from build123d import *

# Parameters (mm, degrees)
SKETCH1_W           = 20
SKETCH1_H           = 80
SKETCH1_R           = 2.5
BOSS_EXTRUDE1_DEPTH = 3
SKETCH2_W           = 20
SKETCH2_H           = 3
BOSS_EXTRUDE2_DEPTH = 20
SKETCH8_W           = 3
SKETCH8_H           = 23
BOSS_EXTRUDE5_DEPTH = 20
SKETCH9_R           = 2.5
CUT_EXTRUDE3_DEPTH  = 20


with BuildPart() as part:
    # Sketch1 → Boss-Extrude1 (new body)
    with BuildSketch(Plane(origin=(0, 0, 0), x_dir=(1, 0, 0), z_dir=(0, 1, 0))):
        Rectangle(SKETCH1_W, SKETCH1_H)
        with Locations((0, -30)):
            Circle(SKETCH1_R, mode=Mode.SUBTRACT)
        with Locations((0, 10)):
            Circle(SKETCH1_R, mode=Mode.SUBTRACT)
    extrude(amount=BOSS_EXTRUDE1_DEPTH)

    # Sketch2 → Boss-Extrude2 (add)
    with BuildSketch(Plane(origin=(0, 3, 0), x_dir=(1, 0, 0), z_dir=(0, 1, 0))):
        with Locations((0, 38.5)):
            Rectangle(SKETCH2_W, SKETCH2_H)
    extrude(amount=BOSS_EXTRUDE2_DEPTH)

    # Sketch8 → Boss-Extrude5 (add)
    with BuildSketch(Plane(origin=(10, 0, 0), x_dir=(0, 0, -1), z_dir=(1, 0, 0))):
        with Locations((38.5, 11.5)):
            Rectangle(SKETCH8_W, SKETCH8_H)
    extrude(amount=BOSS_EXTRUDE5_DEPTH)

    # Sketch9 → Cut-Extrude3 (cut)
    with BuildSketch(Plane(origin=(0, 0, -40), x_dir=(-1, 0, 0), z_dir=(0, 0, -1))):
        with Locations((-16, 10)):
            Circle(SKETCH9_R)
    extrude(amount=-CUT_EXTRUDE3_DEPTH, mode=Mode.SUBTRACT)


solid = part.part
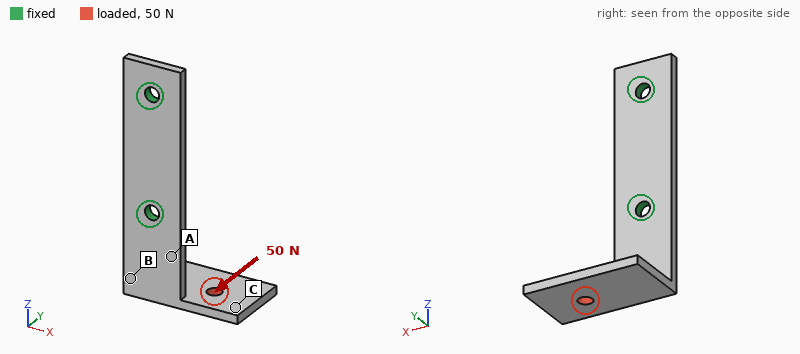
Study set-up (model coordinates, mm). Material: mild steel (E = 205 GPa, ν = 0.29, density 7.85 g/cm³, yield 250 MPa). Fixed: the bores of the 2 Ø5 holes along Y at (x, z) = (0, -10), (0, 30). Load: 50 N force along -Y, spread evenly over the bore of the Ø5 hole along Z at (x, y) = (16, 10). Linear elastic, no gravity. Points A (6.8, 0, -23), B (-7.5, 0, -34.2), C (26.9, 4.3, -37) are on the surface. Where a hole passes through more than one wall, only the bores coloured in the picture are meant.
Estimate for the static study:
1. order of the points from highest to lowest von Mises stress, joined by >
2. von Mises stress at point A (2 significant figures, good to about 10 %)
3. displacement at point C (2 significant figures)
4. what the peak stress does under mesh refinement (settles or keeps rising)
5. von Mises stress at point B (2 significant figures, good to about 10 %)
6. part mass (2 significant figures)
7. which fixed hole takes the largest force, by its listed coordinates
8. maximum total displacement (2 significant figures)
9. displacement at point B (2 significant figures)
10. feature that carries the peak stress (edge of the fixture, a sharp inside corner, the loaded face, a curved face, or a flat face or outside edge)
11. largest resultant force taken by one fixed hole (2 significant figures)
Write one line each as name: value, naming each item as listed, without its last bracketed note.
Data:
order of the points from highest to lowest von Mises stress, joined by >: A > B > C
von Mises stress at point A: 34 MPa
displacement at point C: 0.074 mm
what the peak stress does under mesh refinement: keeps rising
von Mises stress at point B: 20 MPa
part mass: 57 g
which fixed hole takes the largest force, by its listed coordinates: (0, -10)
maximum total displacement: 0.10 mm
displacement at point B: 0.019 mm
feature that carries the peak stress: edge of the fixture
largest resultant force taken by one fixed hole: 52 N
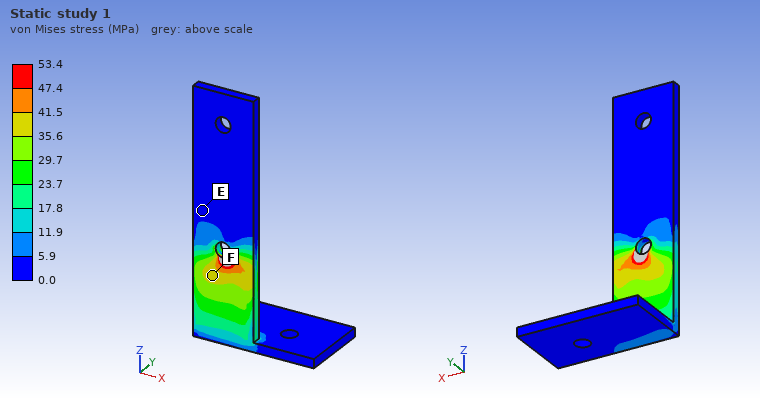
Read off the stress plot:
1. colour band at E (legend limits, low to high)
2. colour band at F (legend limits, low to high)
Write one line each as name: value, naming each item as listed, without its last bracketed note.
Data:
colour band at E: 0.0 to 5.9 MPa
colour band at F: 35.6 to 41.5 MPa
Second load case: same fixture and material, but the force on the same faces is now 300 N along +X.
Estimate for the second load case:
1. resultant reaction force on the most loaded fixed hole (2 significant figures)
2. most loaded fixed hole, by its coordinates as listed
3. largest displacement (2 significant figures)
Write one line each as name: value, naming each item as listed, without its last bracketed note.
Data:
resultant reaction force on the most loaded fixed hole: 430 N
most loaded fixed hole, by its coordinates as listed: (0, -10)
largest displacement: 0.18 mm
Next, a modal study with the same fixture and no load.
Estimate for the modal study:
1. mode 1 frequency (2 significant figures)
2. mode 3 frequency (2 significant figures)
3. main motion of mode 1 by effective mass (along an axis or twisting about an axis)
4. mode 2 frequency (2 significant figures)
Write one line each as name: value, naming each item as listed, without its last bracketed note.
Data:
mode 1 frequency: 920 Hz
mode 3 frequency: 2700 Hz
main motion of mode 1 by effective mass: along Y
mode 2 frequency: 1500 Hz
